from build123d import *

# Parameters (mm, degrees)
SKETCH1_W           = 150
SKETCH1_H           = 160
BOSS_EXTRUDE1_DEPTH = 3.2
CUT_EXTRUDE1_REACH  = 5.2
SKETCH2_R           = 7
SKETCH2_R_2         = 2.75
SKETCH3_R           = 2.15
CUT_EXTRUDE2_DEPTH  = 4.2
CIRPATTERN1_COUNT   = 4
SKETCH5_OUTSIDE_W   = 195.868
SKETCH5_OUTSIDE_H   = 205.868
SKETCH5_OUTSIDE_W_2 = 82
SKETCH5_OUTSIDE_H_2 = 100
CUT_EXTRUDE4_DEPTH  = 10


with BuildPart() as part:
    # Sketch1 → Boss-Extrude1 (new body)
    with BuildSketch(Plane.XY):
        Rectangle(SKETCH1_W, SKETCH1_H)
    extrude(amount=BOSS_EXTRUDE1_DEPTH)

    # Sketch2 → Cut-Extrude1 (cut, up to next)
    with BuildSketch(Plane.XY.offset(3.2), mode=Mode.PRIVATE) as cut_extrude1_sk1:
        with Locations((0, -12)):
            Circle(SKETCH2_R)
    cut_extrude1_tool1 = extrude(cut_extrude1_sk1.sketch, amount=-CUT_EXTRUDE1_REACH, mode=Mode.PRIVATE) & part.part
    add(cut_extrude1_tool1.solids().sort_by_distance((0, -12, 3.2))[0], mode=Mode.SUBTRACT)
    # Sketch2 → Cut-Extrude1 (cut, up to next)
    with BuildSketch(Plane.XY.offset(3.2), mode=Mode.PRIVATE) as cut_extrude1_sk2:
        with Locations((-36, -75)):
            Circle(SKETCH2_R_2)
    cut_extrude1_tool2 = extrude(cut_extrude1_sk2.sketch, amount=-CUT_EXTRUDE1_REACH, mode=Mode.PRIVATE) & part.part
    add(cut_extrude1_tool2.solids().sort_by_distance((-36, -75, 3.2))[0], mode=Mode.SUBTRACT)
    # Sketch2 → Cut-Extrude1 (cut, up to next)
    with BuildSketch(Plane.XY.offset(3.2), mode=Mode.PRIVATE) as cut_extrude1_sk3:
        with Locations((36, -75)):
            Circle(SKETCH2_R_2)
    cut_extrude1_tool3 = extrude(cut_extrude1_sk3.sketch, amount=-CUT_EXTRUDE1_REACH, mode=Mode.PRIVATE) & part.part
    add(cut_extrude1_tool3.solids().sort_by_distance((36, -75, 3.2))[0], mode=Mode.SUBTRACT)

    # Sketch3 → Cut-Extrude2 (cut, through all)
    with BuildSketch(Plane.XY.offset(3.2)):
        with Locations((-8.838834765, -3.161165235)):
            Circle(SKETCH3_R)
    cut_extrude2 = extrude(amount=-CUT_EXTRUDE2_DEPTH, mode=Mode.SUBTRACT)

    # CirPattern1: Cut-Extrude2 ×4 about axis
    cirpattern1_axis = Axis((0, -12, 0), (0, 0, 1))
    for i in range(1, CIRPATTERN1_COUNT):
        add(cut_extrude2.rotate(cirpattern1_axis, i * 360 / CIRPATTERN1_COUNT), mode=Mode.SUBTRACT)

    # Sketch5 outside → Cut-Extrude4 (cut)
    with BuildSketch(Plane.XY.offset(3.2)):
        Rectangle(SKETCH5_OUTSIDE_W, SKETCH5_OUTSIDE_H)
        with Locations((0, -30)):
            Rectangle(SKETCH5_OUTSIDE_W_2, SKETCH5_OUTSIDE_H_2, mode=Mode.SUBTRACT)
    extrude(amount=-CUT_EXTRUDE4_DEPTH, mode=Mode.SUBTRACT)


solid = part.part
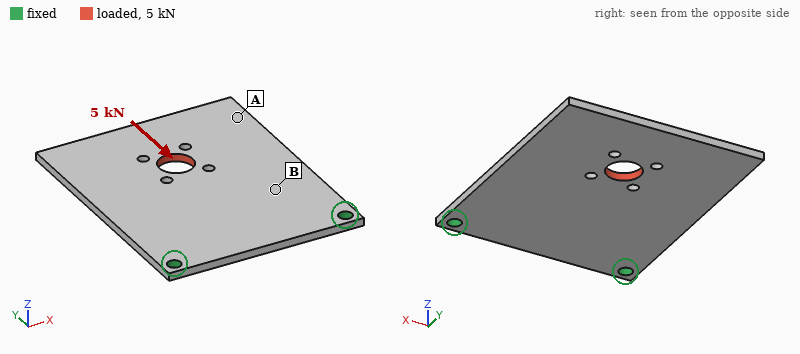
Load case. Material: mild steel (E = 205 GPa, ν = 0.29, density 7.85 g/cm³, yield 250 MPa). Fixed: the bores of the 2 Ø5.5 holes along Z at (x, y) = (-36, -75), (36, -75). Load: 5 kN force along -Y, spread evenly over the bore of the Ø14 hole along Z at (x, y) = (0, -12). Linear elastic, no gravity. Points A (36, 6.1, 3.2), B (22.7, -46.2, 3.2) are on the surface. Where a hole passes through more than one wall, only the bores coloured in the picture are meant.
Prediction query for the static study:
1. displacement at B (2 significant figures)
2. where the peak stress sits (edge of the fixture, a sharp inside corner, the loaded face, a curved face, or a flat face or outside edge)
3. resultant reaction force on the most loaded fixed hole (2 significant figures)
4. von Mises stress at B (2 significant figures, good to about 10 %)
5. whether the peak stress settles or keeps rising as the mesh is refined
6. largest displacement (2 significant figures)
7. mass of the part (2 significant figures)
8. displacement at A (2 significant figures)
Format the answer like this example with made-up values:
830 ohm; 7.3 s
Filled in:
6.3 µm; edge of the fixture; 2.6 kN; 25 MPa; keeps rising; 14 µm; 200 g; 8.2 µm
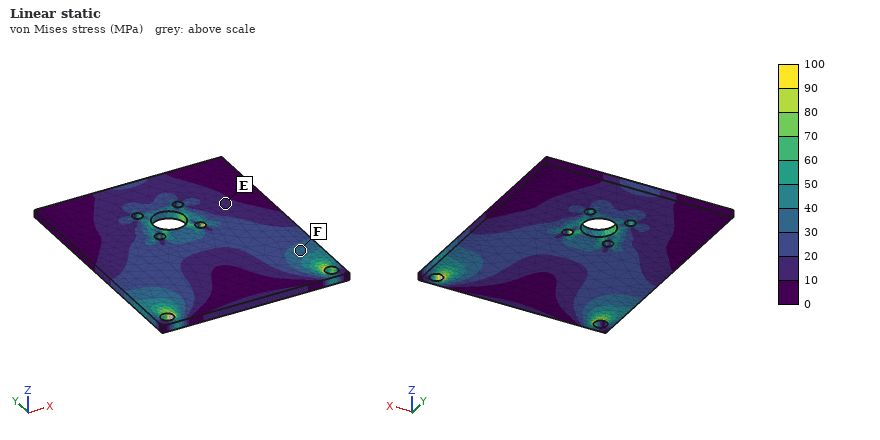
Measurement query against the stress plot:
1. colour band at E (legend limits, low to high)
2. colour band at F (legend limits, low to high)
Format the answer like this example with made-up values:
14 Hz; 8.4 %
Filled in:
10 to 20 MPa; 30 to 40 MPa
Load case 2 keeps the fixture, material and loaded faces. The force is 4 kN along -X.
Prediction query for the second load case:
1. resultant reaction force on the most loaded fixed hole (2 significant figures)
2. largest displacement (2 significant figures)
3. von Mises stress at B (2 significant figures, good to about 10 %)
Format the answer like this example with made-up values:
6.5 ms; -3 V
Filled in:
4.0 kN; 40 µm; 35 MPa
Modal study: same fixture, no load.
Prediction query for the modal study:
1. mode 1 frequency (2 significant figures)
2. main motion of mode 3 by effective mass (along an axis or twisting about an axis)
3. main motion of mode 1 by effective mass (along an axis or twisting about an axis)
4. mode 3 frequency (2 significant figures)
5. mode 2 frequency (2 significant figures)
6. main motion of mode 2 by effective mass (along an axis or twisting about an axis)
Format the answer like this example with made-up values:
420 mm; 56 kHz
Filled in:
250 Hz; along Z; along Z; 1600 Hz; 810 Hz; twisting about Y
